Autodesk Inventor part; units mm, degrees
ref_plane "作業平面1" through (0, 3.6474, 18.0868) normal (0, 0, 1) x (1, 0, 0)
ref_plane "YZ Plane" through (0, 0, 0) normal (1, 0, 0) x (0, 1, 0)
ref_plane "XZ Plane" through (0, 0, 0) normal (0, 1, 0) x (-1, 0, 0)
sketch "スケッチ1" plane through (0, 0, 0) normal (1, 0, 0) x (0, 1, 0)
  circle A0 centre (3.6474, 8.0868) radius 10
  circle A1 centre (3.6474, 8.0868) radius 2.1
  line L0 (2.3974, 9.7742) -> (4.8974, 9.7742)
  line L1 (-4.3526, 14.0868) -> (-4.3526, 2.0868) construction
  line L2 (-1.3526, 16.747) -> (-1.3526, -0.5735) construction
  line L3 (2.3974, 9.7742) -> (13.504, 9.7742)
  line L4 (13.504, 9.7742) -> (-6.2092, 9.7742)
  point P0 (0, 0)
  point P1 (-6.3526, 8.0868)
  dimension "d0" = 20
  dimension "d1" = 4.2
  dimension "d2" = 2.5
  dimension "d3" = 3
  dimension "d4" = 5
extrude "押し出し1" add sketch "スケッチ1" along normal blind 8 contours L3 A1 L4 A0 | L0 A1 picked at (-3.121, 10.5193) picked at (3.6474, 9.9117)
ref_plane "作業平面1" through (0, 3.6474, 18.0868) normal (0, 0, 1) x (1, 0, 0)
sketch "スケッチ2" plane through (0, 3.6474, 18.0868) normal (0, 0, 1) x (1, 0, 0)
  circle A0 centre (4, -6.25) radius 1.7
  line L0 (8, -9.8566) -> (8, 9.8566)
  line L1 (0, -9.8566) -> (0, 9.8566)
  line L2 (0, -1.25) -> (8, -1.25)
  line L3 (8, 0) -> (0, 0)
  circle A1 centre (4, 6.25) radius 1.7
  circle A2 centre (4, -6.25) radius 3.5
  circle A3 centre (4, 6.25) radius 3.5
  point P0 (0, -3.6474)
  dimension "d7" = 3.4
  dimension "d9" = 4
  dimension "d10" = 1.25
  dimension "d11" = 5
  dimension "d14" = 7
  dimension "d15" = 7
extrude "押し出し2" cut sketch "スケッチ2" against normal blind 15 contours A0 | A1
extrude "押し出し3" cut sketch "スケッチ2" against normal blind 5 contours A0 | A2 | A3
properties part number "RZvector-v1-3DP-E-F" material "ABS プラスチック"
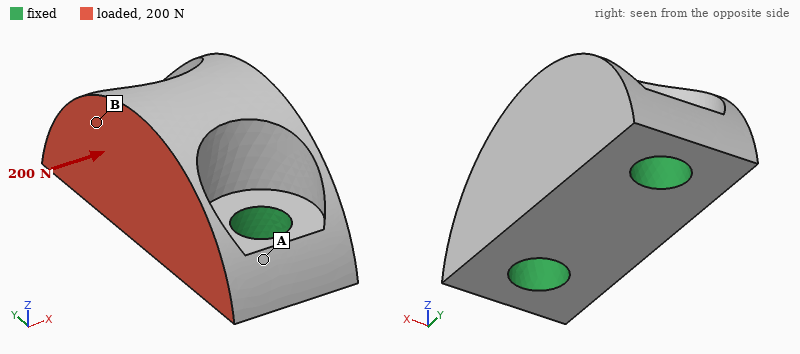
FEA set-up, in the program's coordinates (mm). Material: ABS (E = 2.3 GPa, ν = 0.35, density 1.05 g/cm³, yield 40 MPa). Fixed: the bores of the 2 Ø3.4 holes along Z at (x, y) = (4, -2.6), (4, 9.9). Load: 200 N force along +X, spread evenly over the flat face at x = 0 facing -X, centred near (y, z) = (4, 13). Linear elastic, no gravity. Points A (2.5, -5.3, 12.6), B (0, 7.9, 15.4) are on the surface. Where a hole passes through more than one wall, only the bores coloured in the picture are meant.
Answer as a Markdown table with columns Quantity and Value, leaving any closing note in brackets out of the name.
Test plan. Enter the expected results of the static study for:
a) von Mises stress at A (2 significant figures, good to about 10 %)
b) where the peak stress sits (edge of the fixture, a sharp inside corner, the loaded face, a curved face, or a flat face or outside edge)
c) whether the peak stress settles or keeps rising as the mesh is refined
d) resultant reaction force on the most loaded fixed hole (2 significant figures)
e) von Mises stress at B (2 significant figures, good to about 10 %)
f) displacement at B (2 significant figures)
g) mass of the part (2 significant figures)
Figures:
| Quantity | Value |
|---|---|
| von Mises stress at A | 3.4 MPa |
| where the peak stress sits | edge of the fixture |
| whether the peak stress settles or keeps rising as the mesh is refined | keeps rising |
| resultant reaction force on the most loaded fixed hole | 100 N |
| von Mises stress at B | 8.6 MPa |
| displacement at B | 51 µm |
| mass of the part | 0.77 g |
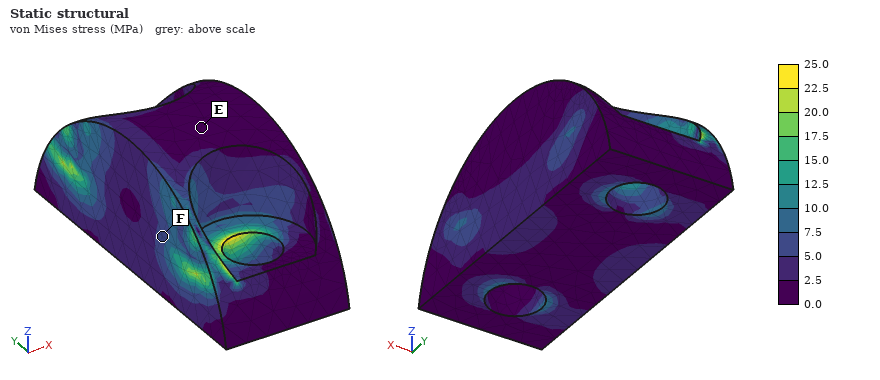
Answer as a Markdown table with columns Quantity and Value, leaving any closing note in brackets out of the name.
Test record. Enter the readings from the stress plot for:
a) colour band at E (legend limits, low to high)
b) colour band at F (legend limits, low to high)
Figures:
| Quantity | Value |
|---|---|
| colour band at E | 0.0 to 2.5 MPa |
| colour band at F | 5.0 to 7.5 MPa |
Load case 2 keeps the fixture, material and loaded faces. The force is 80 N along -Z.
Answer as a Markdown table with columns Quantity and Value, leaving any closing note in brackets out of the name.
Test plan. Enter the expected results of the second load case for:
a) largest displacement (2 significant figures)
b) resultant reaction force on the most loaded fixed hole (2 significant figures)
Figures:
| Quantity | Value |
|---|---|
| largest displacement | 29 µm |
| resultant reaction force on the most loaded fixed hole | 41 N |
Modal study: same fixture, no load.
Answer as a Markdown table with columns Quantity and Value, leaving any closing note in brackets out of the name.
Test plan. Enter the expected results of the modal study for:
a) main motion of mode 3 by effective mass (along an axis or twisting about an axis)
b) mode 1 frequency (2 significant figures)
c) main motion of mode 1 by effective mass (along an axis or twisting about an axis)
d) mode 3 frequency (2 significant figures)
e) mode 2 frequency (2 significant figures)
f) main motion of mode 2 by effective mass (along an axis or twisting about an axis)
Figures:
| Quantity | Value |
|---|---|
| main motion of mode 3 by effective mass | along Y |
| mode 1 frequency | 13 kHz |
| main motion of mode 1 by effective mass | along X |
| mode 3 frequency | 25 kHz |
| mode 2 frequency | 23 kHz |
| main motion of mode 2 by effective mass | along Z |
